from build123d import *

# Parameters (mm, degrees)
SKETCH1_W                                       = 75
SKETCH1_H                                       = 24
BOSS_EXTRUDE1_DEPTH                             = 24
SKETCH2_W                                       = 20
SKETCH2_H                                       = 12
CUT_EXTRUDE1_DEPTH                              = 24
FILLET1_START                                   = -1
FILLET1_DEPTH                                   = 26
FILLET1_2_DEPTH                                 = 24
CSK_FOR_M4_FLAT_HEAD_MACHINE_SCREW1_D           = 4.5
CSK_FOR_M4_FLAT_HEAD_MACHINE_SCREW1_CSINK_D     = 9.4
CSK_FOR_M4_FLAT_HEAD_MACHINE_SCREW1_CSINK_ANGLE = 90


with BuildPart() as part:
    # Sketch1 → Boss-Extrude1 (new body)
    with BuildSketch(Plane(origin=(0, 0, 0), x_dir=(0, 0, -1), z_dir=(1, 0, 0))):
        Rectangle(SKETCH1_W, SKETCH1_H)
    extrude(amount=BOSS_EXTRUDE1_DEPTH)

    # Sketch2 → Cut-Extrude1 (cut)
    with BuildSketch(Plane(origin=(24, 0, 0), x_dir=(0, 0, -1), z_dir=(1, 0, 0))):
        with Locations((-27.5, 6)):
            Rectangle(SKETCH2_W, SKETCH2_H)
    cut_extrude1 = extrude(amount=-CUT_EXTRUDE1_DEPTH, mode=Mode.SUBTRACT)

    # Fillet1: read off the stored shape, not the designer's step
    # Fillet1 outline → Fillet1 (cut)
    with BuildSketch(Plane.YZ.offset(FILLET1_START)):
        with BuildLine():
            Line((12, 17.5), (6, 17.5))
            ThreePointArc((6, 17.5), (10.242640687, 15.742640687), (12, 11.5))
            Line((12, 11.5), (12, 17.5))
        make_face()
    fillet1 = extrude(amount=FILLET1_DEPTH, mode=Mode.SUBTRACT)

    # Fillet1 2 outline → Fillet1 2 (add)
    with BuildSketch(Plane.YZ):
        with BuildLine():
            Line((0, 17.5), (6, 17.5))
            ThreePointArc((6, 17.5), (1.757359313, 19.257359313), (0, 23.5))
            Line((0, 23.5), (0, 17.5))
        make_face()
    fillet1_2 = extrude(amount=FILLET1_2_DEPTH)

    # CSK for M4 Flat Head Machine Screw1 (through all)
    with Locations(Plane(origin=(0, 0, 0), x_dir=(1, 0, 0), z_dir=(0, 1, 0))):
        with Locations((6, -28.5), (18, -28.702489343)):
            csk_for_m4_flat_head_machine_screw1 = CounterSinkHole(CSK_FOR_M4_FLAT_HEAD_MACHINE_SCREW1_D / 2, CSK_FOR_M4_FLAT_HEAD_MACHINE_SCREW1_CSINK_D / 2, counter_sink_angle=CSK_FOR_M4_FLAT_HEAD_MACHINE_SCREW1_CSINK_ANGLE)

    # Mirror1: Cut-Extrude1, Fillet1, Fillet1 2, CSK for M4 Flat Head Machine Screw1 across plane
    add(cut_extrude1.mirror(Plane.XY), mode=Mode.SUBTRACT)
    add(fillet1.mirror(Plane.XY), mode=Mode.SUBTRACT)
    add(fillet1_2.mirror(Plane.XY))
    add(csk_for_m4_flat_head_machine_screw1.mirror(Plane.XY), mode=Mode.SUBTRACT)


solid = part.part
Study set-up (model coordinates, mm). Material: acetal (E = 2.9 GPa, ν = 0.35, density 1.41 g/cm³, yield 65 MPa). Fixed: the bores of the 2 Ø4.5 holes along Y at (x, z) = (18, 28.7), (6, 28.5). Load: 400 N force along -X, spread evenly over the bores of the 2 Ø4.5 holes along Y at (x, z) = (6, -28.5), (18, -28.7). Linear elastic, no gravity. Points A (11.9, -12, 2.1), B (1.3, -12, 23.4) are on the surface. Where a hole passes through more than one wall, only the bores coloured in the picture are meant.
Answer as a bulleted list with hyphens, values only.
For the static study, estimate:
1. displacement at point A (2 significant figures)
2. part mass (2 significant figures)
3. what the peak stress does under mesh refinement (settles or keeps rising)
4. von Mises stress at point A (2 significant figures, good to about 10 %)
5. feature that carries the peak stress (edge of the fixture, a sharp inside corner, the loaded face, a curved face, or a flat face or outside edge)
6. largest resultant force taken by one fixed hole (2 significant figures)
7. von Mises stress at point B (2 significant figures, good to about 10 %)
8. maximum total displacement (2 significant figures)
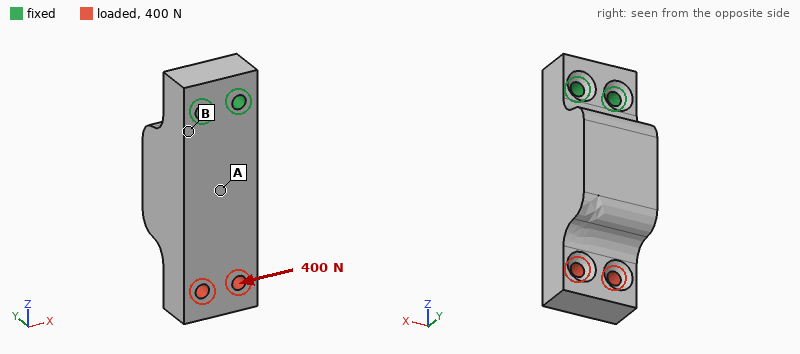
- 0.24 mm
- 43 g
- keeps rising
- 5.0 MPa
- edge of the fixture
- 1.6 kN
- 11 MPa
- 0.85 mm
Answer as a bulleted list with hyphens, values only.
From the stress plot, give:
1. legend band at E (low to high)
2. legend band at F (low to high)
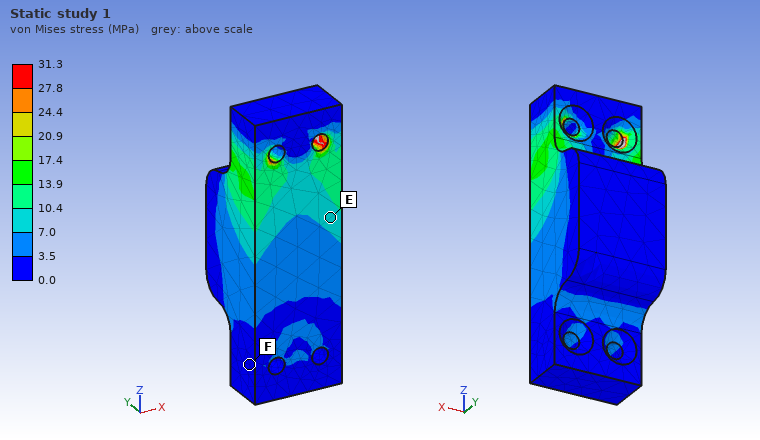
- 7.0 to 10.4 MPa
- 0.0 to 3.5 MPa
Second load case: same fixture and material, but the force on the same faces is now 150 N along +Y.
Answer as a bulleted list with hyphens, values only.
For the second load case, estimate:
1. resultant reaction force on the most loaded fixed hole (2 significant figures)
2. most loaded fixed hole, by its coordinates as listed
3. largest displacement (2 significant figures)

- 81 N
- (6, 28.5)
- 0.80 mm
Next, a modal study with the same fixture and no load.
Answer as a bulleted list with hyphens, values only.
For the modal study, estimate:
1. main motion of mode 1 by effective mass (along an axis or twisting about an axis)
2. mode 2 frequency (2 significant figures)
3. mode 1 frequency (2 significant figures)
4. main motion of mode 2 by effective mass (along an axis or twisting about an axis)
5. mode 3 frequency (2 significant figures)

- along Y
- 1100 Hz
- 630 Hz
- along X
- 2400 Hz
